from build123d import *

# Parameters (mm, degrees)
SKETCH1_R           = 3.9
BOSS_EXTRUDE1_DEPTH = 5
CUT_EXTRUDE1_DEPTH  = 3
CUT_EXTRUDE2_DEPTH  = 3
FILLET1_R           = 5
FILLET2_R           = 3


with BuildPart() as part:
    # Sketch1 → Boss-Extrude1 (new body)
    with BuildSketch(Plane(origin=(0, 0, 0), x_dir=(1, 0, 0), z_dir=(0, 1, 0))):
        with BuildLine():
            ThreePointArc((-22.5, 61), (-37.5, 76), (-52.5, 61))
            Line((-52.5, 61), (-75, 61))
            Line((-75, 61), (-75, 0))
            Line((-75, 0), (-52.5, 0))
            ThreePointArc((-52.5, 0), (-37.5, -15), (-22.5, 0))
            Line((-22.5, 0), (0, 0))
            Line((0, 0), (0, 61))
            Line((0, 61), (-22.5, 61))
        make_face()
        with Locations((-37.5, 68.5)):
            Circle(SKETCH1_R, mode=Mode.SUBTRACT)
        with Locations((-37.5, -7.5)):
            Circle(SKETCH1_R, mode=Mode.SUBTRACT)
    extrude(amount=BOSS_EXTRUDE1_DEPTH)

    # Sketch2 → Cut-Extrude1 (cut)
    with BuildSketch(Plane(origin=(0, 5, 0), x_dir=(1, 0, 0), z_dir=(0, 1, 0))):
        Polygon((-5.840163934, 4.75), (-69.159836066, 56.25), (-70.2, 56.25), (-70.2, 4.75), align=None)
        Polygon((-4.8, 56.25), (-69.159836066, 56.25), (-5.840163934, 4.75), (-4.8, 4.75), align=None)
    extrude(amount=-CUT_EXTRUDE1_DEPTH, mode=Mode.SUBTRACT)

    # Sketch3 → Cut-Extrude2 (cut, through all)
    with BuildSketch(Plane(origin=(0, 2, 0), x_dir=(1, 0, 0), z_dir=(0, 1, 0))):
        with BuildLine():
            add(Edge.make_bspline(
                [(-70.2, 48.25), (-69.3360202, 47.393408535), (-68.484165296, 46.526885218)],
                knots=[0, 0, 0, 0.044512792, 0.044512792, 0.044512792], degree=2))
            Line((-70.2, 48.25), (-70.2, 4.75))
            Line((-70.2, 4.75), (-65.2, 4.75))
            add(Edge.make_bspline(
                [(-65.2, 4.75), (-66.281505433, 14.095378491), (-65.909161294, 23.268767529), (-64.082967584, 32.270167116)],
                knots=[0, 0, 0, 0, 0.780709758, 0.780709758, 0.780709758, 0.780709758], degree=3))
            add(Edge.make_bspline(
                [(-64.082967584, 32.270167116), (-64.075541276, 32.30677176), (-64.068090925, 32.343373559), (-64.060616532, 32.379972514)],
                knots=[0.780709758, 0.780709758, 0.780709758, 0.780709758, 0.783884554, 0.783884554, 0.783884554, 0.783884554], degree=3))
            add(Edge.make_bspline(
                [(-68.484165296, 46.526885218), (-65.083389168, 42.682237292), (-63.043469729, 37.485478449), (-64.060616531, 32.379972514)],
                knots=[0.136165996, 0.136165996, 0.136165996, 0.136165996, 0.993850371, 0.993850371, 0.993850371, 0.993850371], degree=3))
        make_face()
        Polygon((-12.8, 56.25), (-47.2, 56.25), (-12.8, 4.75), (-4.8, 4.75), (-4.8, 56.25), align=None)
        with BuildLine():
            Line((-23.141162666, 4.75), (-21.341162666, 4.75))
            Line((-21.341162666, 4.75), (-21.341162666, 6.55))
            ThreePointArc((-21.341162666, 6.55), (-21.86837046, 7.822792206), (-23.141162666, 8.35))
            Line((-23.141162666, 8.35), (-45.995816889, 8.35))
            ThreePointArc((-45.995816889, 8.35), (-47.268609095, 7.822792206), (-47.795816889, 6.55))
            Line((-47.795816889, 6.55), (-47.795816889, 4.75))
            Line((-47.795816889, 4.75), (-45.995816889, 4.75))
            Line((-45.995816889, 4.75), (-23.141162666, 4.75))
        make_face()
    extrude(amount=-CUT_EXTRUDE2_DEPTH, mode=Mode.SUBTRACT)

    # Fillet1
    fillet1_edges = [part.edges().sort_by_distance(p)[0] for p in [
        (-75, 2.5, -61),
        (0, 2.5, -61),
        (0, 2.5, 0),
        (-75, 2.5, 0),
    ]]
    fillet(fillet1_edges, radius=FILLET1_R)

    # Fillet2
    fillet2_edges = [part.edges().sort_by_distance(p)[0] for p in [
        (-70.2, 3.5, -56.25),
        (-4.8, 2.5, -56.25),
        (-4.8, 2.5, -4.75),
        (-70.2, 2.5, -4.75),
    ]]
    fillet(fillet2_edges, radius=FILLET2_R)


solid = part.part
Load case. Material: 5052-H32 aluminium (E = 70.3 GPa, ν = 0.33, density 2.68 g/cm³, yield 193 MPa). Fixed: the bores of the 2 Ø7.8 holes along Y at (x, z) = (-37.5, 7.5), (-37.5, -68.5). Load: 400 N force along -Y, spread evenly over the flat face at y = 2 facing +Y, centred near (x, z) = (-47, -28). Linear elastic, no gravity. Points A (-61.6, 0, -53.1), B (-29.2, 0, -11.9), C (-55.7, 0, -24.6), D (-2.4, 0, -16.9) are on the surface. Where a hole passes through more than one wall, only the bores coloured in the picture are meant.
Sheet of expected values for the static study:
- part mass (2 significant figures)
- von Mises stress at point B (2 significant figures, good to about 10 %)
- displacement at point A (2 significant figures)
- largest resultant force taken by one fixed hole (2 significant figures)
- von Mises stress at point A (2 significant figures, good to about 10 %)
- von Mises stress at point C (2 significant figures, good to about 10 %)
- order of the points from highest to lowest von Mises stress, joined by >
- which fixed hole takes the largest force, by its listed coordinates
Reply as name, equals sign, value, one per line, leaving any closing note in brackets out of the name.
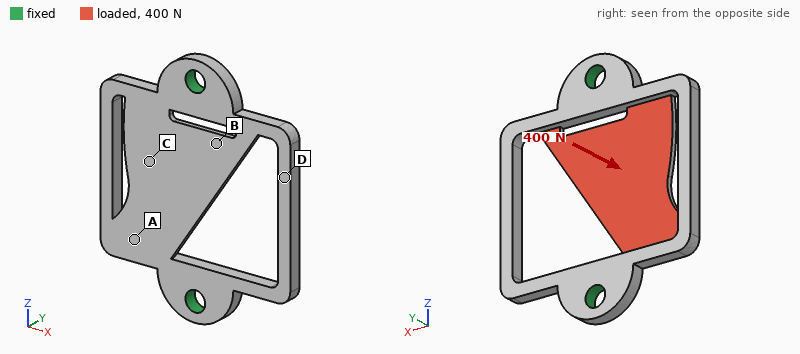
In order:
part mass = 34 g
von Mises stress at point B = 21 MPa
displacement at point A = 0.065 mm
largest resultant force taken by one fixed hole = 280 N
von Mises stress at point A = 32 MPa
von Mises stress at point C = 47 MPa
order of the points from highest to lowest von Mises stress, joined by > = C > A > B > D
which fixed hole takes the largest force, by its listed coordinates = (-37.5, 7.5)
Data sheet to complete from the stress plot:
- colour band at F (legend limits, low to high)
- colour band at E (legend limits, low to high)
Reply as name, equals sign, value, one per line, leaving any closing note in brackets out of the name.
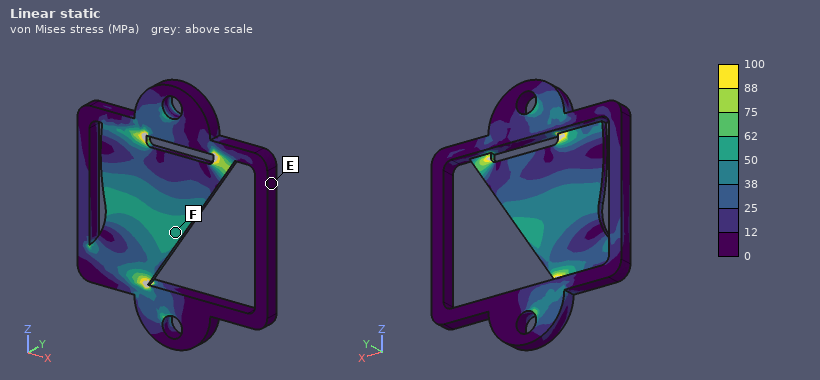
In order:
colour band at F = 50 to 62 MPa
colour band at E = 0 to 12 MPa
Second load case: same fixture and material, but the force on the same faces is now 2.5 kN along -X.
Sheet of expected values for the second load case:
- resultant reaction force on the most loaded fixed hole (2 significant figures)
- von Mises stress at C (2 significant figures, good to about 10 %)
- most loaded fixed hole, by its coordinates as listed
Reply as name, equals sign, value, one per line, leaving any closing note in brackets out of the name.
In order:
resultant reaction force on the most loaded fixed hole = 1.5 kN
von Mises stress at C = 21 MPa
most loaded fixed hole, by its coordinates as listed = (-37.5, 7.5)
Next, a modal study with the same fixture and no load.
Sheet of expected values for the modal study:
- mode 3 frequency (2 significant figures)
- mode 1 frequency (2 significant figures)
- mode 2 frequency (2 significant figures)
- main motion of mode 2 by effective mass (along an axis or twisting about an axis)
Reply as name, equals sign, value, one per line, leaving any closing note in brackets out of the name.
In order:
mode 3 frequency = 2800 Hz
mode 1 frequency = 2000 Hz
mode 2 frequency = 2200 Hz
main motion of mode 2 by effective mass = along Y
